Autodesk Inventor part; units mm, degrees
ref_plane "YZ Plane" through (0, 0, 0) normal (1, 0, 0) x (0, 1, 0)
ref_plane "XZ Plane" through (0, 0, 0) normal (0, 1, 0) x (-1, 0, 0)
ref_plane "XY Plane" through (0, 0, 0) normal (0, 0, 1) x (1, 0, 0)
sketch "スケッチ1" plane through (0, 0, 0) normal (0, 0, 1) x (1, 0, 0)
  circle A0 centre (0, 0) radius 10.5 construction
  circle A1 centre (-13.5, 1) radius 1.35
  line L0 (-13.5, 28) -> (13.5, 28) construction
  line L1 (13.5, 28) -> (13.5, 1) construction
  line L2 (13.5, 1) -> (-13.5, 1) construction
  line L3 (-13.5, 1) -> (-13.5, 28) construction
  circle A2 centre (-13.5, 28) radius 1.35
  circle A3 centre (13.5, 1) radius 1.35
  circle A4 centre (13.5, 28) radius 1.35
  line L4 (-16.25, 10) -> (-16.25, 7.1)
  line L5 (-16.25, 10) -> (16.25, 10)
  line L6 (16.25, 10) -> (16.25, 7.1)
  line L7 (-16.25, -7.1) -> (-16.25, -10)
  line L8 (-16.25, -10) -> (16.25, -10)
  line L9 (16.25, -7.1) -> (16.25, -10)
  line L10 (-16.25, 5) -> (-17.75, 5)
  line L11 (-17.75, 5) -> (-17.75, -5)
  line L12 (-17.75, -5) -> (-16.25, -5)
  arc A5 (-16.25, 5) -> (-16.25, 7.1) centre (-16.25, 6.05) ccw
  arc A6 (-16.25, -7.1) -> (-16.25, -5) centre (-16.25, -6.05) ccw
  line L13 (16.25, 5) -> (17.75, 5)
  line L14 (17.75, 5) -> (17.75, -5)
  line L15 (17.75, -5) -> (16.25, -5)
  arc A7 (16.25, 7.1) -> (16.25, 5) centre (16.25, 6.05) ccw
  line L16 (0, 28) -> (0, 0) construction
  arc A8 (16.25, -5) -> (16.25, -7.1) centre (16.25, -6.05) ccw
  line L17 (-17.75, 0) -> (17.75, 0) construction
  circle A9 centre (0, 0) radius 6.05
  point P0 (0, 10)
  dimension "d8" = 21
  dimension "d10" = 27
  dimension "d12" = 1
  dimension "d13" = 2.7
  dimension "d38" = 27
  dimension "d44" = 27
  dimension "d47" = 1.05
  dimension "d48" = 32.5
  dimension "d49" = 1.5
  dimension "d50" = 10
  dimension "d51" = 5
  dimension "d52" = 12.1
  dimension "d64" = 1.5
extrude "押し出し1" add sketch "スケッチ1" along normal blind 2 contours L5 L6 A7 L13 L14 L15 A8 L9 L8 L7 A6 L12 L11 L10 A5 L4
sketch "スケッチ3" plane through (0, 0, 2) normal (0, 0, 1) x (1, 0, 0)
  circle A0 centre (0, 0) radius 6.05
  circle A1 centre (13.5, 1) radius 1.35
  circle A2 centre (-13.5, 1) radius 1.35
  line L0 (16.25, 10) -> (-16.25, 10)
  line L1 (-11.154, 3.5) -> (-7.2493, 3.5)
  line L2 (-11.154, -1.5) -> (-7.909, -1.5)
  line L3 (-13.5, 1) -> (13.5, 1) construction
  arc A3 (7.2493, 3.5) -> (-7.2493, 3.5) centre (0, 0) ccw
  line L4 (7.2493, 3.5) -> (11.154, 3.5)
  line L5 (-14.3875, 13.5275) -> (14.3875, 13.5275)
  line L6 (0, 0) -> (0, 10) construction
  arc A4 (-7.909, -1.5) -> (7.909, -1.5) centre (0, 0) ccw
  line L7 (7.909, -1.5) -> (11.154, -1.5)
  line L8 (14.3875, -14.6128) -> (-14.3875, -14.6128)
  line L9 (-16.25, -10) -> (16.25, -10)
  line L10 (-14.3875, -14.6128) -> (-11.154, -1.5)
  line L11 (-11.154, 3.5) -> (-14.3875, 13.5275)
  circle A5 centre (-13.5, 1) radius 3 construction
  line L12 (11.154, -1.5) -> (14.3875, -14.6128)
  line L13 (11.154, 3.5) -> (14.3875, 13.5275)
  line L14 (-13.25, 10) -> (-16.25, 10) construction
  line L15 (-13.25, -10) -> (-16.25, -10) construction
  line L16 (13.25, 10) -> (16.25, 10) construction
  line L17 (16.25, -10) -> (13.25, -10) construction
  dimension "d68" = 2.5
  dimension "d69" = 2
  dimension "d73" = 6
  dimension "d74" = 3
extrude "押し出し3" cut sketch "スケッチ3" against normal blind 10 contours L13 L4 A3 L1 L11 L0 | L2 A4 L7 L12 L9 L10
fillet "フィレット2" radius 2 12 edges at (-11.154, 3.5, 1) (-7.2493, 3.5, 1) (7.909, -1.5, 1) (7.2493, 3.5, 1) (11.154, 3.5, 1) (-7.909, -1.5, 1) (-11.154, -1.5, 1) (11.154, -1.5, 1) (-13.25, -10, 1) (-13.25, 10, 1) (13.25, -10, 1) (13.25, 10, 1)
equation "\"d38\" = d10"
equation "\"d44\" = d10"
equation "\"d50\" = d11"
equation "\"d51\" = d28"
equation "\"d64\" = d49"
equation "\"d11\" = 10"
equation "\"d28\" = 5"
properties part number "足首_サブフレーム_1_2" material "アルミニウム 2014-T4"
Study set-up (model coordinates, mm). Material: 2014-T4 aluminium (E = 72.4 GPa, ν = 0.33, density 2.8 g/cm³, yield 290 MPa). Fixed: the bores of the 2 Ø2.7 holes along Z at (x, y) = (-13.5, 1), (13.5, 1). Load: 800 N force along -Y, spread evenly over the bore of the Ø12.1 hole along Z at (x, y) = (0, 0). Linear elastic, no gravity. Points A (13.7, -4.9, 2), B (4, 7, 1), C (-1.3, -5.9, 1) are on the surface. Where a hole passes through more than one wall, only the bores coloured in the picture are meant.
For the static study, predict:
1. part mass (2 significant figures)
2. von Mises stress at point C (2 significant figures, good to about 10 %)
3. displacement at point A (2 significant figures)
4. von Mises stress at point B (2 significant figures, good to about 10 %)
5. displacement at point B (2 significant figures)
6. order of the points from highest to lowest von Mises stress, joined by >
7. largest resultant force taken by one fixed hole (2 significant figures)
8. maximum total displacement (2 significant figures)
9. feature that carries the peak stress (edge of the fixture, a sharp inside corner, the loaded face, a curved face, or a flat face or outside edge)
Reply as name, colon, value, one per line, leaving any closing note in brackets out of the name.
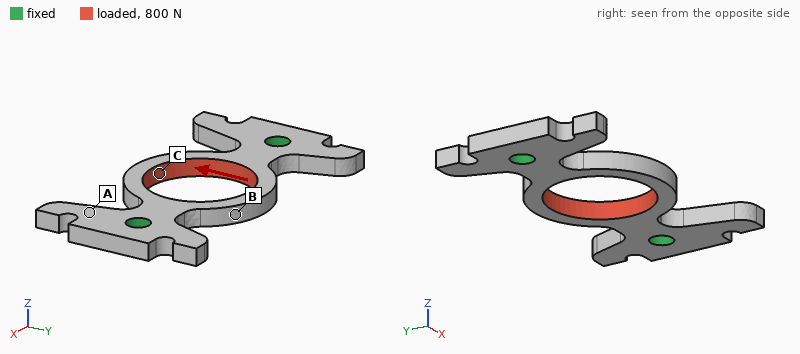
part mass: 1.7 g
von Mises stress at point C: 55 MPa
displacement at point A: 6.7 µm
von Mises stress at point B: 39 MPa
displacement at point B: 21 µm
order of the points from highest to lowest von Mises stress, joined by >: C > B > A
largest resultant force taken by one fixed hole: 400 N
maximum total displacement: 21 µm
feature that carries the peak stress: edge of the fixture
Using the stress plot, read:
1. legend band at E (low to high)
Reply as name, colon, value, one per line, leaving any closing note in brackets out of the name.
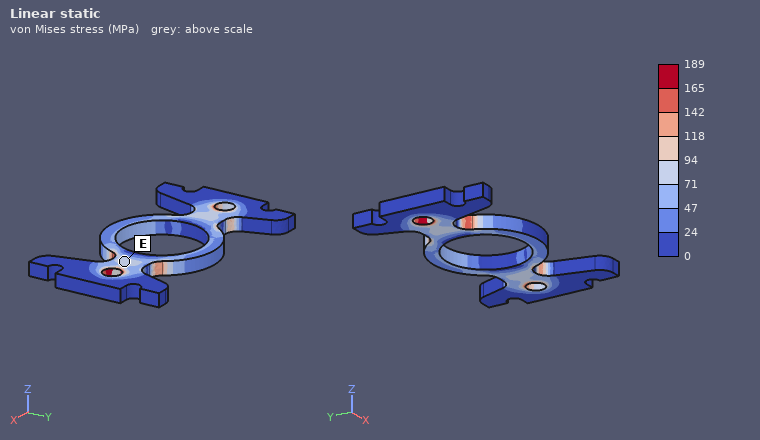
legend band at E: 71 to 94 MPa
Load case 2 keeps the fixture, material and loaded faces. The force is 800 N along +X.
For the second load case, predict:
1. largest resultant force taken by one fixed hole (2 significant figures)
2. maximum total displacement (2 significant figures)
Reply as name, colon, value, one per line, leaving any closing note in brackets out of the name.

largest resultant force taken by one fixed hole: 400 N
maximum total displacement: 26 µm
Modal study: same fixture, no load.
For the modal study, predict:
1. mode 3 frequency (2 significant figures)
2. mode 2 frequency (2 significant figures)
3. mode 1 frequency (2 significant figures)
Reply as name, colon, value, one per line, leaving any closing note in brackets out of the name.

mode 3 frequency: 21 kHz
mode 2 frequency: 14 kHz
mode 1 frequency: 11 kHz
